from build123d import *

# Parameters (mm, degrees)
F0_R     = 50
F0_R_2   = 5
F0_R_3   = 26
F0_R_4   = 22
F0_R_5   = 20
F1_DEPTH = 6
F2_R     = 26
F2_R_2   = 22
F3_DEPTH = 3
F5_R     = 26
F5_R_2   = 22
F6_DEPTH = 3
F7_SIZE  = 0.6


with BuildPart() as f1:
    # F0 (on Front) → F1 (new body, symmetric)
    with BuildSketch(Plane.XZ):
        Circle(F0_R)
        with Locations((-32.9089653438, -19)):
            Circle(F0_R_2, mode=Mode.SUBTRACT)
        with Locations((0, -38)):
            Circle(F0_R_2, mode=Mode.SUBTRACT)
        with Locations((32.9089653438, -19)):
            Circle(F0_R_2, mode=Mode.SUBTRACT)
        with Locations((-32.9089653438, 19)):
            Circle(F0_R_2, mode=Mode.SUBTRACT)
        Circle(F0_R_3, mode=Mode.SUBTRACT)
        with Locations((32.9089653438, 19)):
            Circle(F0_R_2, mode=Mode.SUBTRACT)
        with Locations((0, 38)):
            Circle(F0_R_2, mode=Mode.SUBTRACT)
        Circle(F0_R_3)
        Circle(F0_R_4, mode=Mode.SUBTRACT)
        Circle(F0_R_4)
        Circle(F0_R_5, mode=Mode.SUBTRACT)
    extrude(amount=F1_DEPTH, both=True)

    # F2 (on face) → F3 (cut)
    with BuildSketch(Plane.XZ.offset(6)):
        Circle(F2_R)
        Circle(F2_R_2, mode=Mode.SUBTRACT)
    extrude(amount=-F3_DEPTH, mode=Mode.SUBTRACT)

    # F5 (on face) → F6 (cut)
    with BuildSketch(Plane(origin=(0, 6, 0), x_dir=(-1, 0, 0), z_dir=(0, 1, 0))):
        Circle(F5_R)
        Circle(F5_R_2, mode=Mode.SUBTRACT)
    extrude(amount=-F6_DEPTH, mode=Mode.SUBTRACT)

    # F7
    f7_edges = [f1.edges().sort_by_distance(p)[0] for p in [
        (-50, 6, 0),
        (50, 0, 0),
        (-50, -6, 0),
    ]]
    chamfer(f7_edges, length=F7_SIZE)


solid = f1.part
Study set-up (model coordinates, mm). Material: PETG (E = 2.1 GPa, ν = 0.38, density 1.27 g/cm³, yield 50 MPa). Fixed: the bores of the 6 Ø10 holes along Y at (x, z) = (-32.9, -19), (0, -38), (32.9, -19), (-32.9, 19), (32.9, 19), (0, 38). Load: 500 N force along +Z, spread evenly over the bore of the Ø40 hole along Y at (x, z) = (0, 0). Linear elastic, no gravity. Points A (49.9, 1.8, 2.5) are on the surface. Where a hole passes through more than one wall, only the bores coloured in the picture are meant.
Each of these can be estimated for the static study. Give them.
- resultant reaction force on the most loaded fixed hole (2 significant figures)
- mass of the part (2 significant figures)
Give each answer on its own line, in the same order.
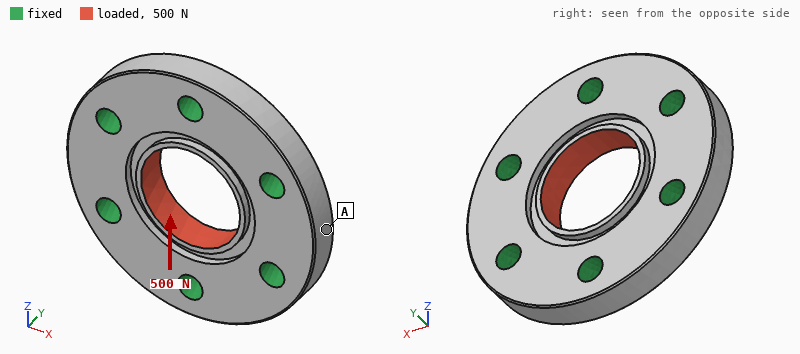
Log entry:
120 N
89 g
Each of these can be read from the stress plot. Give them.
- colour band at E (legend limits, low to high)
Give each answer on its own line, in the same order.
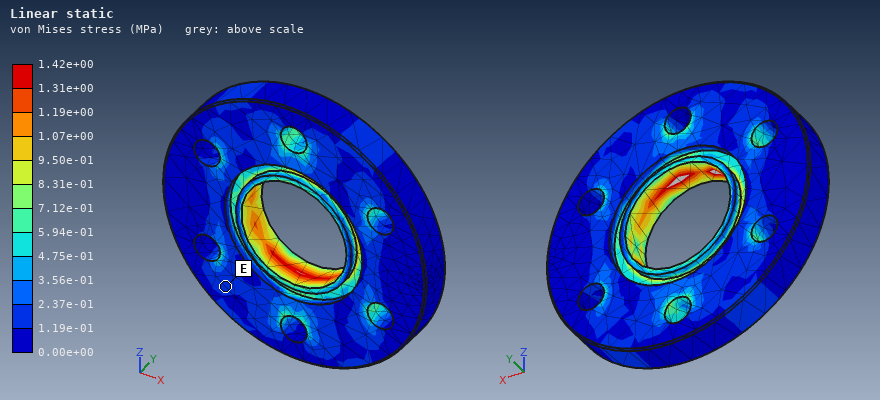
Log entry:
1.19e-01 to 2.37e-01 MPa
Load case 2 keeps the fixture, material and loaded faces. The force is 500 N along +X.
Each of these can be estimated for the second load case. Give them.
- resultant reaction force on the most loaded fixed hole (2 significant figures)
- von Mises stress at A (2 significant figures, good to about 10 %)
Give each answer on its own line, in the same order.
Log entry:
100 N
0.18 MPa
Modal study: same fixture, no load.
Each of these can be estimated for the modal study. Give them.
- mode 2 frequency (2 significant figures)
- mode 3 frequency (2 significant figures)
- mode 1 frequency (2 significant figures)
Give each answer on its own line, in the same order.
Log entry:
6800 Hz
6900 Hz
6800 Hz
